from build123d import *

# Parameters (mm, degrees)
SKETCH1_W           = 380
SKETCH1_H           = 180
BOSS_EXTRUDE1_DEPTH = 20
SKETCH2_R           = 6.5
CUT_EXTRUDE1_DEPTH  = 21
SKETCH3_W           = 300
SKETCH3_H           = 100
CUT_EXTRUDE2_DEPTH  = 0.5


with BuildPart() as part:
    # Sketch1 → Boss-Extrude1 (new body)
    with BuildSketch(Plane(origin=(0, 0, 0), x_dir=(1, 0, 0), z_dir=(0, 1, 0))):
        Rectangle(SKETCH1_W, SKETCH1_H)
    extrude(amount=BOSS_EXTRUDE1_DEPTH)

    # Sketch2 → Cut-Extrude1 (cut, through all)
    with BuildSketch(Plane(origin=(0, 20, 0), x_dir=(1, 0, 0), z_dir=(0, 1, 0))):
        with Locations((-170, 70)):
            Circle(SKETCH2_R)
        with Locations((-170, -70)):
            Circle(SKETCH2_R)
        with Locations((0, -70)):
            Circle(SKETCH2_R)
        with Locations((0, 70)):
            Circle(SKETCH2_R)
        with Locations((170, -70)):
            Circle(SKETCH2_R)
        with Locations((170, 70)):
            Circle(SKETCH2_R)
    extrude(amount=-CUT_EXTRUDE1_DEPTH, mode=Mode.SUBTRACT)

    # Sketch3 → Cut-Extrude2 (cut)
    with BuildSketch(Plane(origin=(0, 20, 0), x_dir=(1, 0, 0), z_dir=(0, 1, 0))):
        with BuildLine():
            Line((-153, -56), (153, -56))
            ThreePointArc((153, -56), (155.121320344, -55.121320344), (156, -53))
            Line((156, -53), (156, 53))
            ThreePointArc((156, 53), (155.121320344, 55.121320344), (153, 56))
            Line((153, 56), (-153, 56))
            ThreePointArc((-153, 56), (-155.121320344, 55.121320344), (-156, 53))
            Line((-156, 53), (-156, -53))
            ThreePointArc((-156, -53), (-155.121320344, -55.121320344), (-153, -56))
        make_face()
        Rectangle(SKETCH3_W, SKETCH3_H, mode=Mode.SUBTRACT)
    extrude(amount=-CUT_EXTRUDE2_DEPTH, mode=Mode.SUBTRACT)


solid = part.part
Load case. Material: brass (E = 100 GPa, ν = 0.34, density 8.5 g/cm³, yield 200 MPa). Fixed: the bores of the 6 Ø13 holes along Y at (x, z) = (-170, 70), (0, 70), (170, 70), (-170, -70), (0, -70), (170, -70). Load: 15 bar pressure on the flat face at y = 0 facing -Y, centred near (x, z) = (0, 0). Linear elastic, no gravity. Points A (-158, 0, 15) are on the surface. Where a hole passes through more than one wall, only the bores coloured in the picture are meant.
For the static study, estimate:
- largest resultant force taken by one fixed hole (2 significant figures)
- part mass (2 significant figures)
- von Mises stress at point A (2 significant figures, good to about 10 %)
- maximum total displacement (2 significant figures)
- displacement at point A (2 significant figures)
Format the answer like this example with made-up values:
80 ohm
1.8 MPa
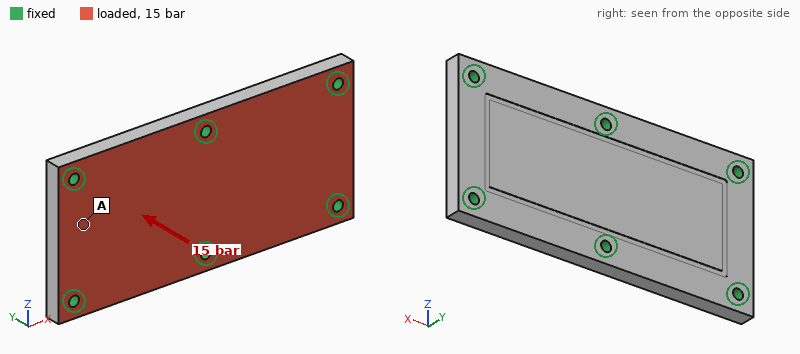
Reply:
24 kN
11 kg
20 MPa
92 µm
47 µm
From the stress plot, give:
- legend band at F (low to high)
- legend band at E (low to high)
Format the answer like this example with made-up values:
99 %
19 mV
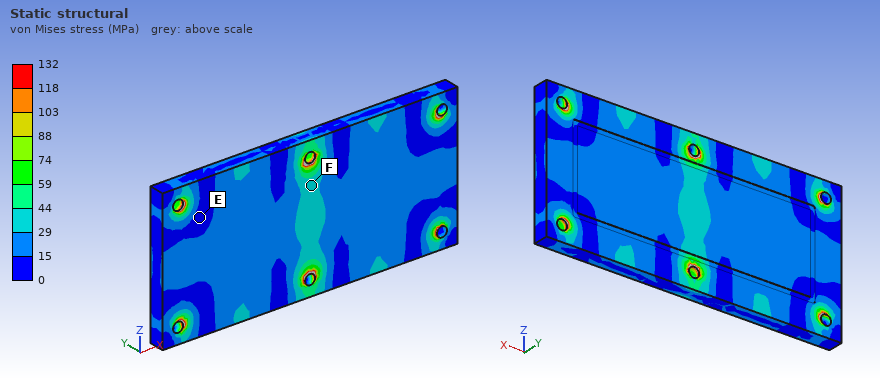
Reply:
29 to 44 MPa
0 to 15 MPa
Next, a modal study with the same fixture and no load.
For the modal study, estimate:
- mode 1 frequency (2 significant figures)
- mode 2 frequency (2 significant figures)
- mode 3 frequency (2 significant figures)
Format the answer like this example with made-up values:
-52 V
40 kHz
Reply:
1800 Hz
1800 Hz
2600 Hz
